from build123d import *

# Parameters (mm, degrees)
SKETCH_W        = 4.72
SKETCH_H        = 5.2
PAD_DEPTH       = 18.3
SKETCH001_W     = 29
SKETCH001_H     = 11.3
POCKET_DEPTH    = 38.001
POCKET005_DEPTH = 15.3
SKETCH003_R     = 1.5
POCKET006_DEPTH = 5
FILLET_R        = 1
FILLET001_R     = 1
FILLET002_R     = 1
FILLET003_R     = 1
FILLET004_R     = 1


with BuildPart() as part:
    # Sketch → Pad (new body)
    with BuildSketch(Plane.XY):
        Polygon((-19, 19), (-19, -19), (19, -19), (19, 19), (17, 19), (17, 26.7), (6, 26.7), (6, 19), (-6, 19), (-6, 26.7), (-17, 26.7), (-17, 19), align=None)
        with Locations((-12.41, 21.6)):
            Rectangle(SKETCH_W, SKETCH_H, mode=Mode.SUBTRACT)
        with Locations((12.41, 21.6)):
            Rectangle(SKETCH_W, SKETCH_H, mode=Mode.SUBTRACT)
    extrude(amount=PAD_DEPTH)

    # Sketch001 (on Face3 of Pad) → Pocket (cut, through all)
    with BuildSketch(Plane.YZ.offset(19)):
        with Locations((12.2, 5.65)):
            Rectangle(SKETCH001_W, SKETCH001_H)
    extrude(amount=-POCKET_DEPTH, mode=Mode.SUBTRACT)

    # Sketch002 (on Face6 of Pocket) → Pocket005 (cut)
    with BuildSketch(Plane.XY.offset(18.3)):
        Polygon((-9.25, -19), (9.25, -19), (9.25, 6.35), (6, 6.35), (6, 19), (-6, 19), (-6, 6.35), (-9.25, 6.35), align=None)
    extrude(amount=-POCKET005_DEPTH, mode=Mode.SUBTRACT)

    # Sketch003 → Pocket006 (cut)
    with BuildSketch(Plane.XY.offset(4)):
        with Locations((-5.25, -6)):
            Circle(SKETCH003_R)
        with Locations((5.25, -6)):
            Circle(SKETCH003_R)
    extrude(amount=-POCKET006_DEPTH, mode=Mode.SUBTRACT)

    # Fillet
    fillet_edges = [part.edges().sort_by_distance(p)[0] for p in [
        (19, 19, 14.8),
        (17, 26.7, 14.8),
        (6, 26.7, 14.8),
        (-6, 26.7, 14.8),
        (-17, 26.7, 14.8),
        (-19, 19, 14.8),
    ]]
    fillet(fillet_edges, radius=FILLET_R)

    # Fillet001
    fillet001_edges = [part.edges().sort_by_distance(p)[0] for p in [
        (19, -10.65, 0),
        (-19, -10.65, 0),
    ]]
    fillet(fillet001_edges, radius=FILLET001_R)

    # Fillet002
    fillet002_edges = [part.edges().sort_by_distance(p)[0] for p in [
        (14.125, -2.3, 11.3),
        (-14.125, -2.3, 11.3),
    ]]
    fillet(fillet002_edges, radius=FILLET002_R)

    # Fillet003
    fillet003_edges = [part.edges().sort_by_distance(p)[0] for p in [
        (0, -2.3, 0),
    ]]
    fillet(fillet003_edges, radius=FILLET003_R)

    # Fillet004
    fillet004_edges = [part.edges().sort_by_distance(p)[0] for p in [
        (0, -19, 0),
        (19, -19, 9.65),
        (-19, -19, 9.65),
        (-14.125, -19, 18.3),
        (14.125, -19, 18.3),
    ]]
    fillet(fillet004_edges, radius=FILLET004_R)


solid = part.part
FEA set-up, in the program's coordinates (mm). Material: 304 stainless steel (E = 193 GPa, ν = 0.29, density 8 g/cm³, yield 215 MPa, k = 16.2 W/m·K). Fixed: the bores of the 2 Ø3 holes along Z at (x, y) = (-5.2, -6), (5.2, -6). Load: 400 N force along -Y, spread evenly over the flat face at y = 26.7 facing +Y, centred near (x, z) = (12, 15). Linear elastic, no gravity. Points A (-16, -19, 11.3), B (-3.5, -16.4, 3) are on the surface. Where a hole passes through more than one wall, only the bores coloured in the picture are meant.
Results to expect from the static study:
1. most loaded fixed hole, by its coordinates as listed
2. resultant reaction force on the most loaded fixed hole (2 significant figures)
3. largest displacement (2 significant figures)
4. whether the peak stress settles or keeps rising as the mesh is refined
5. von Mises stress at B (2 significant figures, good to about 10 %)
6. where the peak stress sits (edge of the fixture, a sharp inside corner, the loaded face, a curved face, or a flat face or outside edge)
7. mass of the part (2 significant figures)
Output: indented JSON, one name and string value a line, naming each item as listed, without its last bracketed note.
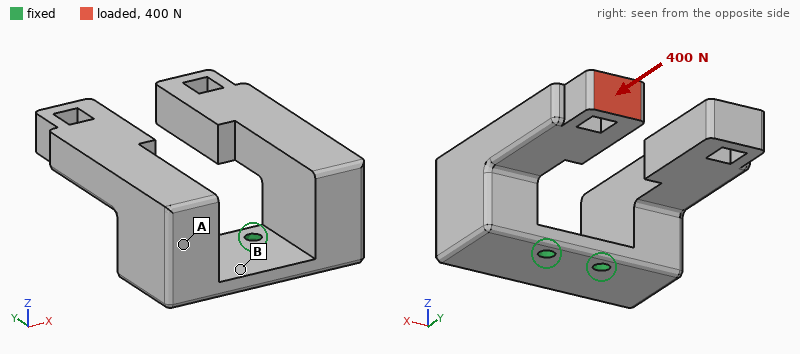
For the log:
{
  "most loaded fixed hole, by its coordinates as listed": "(5.2, -6)",
  "resultant reaction force on the most loaded fixed hole": "540 N",
  "largest displacement": "97 µm",
  "whether the peak stress settles or keeps rising as the mesh is refined": "keeps rising",
  "von Mises stress at B": "43 MPa",
  "where the peak stress sits": "edge of the fixture",
  "mass of the part": "89 g"
}
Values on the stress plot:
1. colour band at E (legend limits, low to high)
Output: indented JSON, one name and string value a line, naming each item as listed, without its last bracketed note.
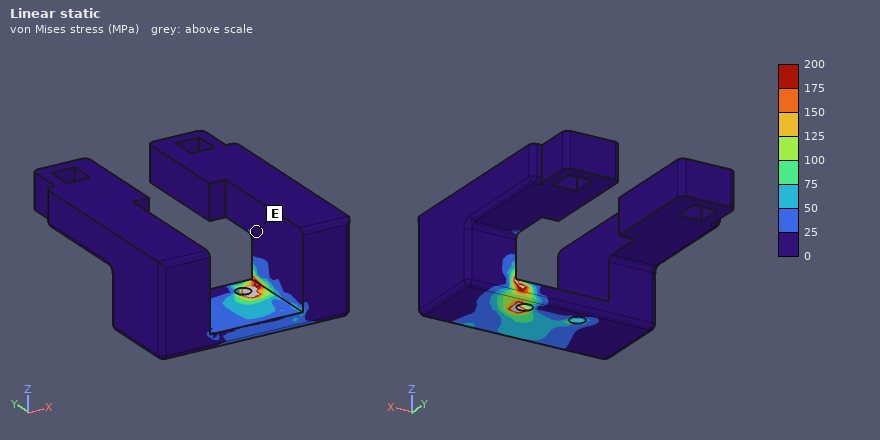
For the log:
{
  "colour band at E": "0 to 25 MPa"
}
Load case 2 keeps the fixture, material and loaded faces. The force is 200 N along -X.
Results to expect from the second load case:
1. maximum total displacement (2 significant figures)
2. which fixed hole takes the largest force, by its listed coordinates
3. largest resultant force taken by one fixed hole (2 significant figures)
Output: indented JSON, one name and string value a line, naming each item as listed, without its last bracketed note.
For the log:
{
  "maximum total displacement": "94 µm",
  "which fixed hole takes the largest force, by its listed coordinates": "(5.2, -6)",
  "largest resultant force taken by one fixed hole": "640 N"
}
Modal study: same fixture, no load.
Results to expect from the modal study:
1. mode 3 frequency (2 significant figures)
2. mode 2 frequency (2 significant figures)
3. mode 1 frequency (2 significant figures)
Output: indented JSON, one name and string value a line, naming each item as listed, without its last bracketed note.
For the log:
{
  "mode 3 frequency": "2000 Hz",
  "mode 2 frequency": "1900 Hz",
  "mode 1 frequency": "1800 Hz"
}
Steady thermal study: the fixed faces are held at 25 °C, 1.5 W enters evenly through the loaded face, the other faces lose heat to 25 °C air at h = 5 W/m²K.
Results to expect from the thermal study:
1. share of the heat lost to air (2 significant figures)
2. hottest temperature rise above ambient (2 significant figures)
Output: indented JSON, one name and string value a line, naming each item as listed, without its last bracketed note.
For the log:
{
  "share of the heat lost to air": "22 %",
  "hottest temperature rise above ambient": "61 K"
}
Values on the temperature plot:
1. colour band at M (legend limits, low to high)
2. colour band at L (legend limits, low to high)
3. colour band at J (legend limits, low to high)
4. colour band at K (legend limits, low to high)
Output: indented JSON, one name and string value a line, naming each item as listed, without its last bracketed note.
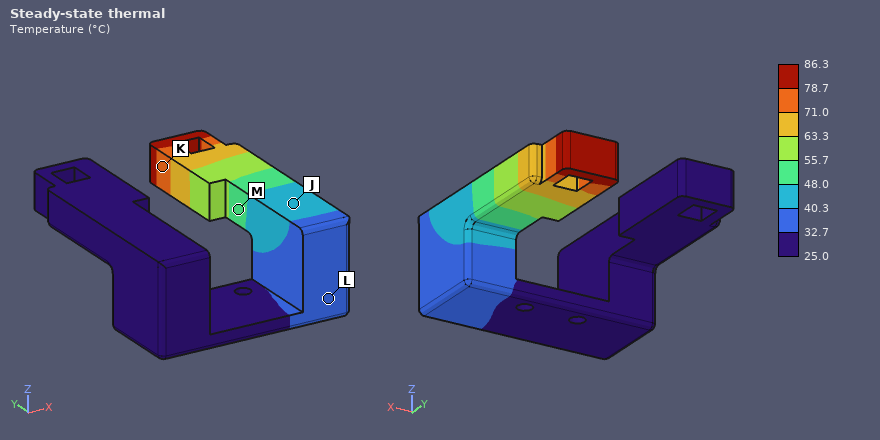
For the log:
{
  "colour band at M": "48.0 to 55.7 °C",
  "colour band at L": "32.7 to 40.3 °C",
  "colour band at J": "40.3 to 48.0 °C",
  "colour band at K": "71.0 to 78.7 °C"
}
